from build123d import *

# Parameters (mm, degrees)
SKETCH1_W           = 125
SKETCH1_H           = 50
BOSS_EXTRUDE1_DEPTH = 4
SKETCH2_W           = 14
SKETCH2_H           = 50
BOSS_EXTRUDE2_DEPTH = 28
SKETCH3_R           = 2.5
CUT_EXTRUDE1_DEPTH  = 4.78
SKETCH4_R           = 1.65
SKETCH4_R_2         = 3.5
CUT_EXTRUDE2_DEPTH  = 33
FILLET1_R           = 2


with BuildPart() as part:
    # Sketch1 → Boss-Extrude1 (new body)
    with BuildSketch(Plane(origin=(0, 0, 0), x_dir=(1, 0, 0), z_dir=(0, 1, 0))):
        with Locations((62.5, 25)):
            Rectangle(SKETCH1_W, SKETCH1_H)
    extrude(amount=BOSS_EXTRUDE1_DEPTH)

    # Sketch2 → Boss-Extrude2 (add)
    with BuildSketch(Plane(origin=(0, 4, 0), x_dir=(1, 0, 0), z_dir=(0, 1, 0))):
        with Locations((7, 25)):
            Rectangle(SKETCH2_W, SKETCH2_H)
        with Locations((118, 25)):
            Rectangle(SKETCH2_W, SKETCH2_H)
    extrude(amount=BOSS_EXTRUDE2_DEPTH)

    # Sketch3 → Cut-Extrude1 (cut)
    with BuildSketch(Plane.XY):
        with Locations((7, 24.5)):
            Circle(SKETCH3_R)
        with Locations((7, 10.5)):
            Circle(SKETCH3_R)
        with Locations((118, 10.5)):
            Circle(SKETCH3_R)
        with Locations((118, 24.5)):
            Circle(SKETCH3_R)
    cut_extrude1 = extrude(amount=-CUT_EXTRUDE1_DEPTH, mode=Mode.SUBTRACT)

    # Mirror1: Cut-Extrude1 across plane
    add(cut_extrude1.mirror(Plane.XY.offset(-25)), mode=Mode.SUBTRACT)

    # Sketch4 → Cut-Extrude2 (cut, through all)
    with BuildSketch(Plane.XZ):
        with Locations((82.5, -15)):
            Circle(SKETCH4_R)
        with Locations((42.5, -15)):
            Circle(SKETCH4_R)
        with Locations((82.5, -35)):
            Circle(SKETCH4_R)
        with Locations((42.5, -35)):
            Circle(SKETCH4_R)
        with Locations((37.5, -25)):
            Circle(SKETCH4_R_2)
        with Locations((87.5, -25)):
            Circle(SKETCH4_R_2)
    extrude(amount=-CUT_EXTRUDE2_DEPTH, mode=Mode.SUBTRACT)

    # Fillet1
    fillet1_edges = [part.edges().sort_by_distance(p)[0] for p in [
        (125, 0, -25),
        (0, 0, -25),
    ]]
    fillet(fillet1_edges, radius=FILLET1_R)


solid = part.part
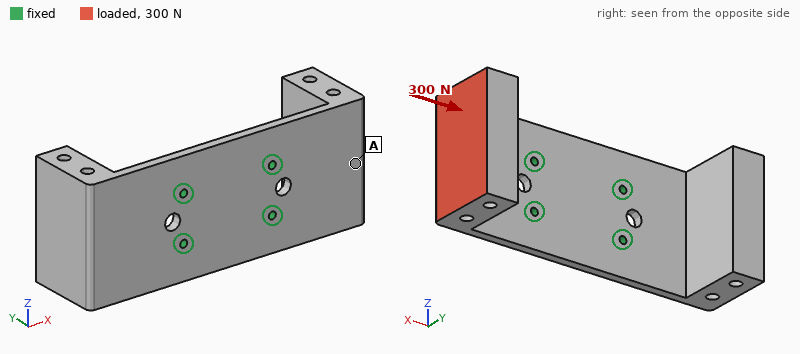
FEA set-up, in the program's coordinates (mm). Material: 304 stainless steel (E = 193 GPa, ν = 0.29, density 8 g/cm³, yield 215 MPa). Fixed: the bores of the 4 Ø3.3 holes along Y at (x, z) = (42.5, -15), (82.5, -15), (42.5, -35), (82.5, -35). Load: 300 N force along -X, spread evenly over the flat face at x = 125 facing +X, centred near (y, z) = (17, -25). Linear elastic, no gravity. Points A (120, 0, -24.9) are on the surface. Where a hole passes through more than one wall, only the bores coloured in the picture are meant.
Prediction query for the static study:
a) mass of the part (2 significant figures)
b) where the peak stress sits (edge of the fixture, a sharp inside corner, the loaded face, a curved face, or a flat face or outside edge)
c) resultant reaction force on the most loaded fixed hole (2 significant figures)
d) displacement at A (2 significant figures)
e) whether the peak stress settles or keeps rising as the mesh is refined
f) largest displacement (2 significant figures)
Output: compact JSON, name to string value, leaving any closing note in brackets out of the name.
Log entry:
{"mass of the part": "500 g", "where the peak stress sits": "edge of the fixture", "resultant reaction force on the most loaded fixed hole": "130 N", "displacement at A": "0.065 mm", "whether the peak stress settles or keeps rising as the mesh is refined": "keeps rising", "largest displacement": "0.11 mm"}
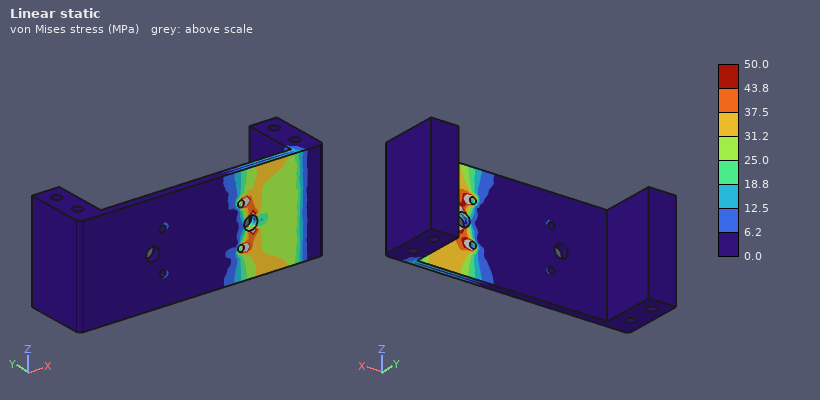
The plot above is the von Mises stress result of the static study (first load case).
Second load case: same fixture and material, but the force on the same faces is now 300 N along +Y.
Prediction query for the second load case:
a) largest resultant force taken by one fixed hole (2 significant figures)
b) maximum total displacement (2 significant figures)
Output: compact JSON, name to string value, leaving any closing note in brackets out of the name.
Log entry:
{"largest resultant force taken by one fixed hole": "190 N", "maximum total displacement": "0.23 mm"}
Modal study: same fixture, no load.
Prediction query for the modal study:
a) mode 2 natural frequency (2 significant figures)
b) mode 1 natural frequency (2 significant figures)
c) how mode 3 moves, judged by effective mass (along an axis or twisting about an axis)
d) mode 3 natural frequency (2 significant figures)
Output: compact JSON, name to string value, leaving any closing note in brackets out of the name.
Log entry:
{"mode 2 natural frequency": "540 Hz", "mode 1 natural frequency": "530 Hz", "how mode 3 moves, judged by effective mass": "along Z", "mode 3 natural frequency": "1200 Hz"}
